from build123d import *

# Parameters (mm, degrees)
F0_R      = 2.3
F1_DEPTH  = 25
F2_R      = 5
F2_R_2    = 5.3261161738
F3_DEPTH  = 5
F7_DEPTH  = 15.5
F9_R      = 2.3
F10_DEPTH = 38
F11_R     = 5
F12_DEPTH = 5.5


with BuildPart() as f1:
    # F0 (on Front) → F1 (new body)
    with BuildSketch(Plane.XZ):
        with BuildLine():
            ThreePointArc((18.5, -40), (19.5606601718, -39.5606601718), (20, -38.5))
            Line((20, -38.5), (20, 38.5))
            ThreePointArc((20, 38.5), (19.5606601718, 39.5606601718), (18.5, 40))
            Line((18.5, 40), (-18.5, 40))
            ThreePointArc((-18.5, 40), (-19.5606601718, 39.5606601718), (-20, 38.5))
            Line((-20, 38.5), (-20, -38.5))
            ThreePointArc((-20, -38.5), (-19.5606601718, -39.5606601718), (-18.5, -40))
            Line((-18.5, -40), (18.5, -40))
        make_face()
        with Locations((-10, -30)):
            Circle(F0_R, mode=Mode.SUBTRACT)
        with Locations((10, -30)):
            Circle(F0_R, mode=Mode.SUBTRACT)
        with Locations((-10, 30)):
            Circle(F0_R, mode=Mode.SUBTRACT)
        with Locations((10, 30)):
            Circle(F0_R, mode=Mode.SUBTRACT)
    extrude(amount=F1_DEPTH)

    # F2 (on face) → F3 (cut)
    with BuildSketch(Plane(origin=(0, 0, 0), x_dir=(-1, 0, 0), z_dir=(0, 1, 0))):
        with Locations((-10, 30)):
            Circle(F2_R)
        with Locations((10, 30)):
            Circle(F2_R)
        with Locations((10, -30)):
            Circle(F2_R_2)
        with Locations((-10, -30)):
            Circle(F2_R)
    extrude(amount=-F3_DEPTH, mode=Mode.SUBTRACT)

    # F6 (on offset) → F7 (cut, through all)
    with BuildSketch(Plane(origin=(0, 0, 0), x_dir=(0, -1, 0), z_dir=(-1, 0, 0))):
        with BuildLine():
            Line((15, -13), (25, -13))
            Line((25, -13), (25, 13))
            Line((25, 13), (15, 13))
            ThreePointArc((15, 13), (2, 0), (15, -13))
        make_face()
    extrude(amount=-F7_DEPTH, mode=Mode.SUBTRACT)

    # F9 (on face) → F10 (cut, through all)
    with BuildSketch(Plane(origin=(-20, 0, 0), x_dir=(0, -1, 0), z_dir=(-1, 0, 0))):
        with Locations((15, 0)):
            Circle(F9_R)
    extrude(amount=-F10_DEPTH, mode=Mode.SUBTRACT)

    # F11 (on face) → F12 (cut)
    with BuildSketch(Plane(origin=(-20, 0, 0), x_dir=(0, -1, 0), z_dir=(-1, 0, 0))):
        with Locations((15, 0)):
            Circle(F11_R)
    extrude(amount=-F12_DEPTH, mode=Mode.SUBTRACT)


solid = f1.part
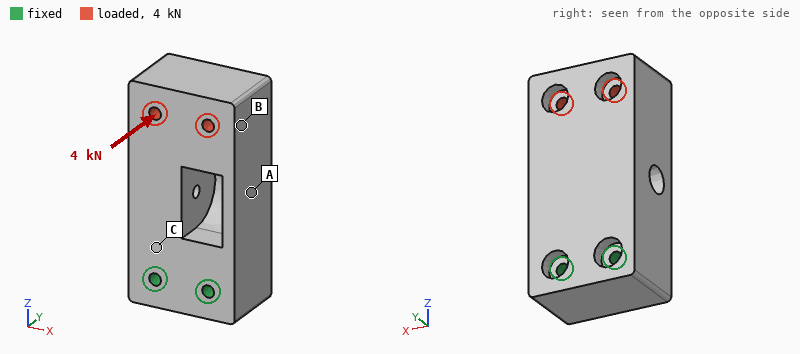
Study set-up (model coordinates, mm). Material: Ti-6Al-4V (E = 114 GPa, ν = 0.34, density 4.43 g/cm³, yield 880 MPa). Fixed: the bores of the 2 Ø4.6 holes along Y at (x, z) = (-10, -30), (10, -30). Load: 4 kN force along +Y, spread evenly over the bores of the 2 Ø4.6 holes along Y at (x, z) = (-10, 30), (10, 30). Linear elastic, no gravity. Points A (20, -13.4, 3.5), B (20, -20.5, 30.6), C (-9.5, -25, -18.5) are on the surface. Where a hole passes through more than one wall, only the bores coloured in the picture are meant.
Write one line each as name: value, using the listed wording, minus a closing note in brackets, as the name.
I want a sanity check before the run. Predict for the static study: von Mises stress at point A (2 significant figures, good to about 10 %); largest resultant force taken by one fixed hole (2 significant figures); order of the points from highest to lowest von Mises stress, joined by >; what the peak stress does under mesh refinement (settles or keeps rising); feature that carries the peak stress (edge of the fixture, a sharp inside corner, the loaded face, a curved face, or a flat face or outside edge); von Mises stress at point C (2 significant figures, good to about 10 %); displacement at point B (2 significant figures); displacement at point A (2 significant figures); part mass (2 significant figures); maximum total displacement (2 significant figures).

von Mises stress at point A: 34 MPa
largest resultant force taken by one fixed hole: 2.0 kN
order of the points from highest to lowest von Mises stress, joined by >: C > A > B
what the peak stress does under mesh refinement: keeps rising
feature that carries the peak stress: edge of the fixture
von Mises stress at point C: 71 MPa
displacement at point B: 0.097 mm
displacement at point A: 0.039 mm
part mass: 300 g
maximum total displacement: 0.12 mm
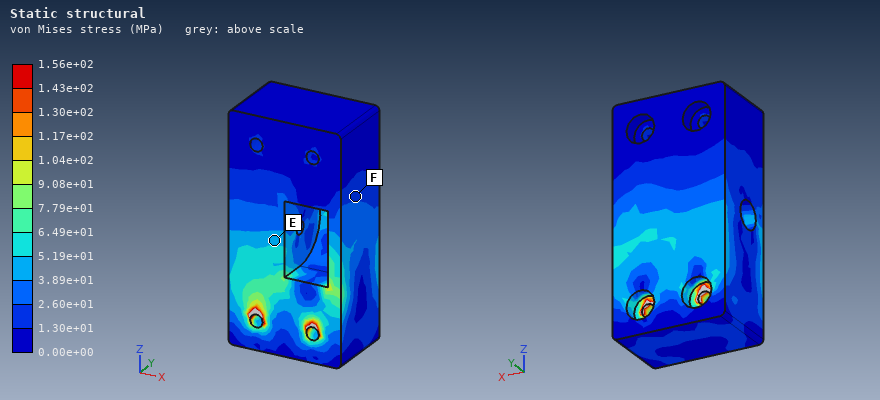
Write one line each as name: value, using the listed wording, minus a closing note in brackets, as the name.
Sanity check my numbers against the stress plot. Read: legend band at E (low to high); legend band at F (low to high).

legend band at E: 3.89e+01 to 5.19e+01 MPa
legend band at F: 1.30e+01 to 2.60e+01 MPa
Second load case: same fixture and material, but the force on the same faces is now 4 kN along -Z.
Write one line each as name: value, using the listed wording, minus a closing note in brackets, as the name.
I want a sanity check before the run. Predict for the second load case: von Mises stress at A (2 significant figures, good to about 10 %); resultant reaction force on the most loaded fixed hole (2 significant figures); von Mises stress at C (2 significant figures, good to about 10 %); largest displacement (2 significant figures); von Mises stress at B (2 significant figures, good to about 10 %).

von Mises stress at A: 11 MPa
resultant reaction force on the most loaded fixed hole: 2.0 kN
von Mises stress at C: 10.0 MPa
largest displacement: 9.7 µm
von Mises stress at B: 2.4 MPa
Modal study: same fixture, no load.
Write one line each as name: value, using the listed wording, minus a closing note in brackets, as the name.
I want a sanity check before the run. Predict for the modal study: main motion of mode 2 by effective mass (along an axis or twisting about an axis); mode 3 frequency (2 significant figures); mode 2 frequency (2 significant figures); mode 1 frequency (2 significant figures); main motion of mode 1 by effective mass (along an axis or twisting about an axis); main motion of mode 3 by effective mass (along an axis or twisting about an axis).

main motion of mode 2 by effective mass: along X
mode 3 frequency: 7900 Hz
mode 2 frequency: 4100 Hz
mode 1 frequency: 3100 Hz
main motion of mode 1 by effective mass: along Y
main motion of mode 3 by effective mass: twisting about Z
